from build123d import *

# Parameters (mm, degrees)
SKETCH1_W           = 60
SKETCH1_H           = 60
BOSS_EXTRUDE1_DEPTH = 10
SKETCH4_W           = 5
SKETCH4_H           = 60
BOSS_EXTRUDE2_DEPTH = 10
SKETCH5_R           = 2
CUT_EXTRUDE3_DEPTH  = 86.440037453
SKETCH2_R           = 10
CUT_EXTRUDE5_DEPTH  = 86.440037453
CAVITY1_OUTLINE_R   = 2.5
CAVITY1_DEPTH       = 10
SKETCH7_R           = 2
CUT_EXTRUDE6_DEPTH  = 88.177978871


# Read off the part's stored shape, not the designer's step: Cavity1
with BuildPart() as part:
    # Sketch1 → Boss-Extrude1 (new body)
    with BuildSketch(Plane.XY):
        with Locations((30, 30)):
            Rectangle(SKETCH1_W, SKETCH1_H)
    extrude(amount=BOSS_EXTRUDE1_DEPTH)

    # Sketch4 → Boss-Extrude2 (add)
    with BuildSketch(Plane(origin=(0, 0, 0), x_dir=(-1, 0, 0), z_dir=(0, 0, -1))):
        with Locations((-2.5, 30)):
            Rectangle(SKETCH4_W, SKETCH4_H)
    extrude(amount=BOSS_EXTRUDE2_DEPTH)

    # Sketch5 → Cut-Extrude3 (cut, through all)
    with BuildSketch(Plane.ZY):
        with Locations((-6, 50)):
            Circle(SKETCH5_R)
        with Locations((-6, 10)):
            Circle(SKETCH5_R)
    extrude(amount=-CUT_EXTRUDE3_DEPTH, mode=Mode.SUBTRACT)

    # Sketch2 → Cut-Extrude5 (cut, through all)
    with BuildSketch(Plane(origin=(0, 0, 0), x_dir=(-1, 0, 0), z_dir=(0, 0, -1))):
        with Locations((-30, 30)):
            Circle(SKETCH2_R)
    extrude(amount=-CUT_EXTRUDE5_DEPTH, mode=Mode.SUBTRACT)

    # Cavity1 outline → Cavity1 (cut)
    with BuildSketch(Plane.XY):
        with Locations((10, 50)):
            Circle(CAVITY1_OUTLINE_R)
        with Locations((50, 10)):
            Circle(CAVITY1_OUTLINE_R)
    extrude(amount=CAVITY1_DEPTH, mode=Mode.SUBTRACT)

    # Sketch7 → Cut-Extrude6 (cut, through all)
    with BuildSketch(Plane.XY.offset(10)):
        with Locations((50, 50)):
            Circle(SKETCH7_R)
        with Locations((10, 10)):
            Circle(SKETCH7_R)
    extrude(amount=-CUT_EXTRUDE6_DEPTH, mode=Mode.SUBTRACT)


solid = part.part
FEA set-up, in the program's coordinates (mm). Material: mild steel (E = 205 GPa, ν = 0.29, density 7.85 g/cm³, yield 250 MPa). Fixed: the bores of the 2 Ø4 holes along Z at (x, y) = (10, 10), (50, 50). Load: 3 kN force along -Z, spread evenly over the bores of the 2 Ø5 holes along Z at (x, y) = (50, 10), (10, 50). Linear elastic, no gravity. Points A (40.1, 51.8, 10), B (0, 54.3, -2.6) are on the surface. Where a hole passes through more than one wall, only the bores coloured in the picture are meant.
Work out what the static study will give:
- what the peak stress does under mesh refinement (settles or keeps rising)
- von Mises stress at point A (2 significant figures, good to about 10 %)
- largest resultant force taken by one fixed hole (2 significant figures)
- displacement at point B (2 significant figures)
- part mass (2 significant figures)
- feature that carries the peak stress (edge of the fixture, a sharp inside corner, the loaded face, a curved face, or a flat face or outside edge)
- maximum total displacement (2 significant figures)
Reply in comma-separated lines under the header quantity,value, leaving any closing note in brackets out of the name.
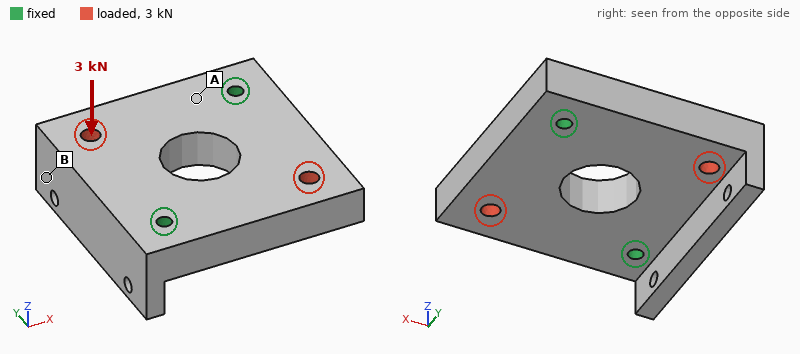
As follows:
quantity,value
what the peak stress does under mesh refinement,keeps rising
von Mises stress at point A,31 MPa
largest resultant force taken by one fixed hole,1.6 kN
displacement at point B,27 µm
part mass,280 g
feature that carries the peak stress,edge of the fixture
maximum total displacement,39 µm
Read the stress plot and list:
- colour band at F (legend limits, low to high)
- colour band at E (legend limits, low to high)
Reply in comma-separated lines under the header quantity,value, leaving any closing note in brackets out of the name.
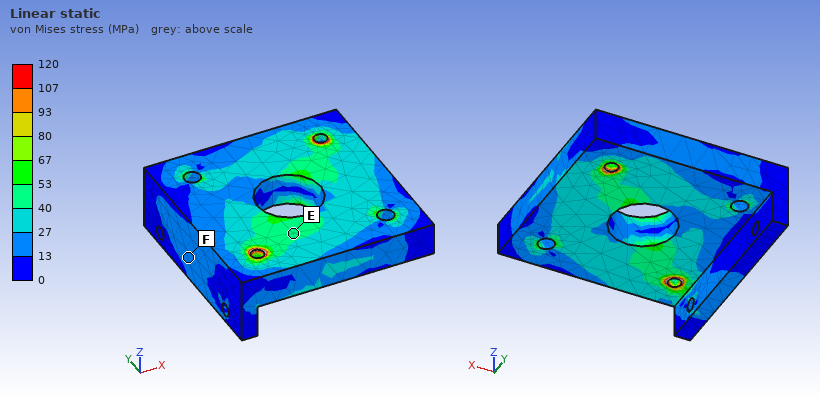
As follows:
quantity,value
colour band at F,13 to 27 MPa
colour band at E,40 to 53 MPa
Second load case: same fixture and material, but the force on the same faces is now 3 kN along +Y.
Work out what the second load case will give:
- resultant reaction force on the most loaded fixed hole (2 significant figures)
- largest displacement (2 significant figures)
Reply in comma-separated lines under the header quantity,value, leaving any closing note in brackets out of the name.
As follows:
quantity,value
resultant reaction force on the most loaded fixed hole,1.5 kN
largest displacement,2.1 µm
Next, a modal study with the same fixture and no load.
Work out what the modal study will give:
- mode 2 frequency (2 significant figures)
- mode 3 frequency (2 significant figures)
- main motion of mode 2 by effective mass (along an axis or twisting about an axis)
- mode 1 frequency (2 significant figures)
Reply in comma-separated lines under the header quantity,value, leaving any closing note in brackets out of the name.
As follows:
quantity,value
mode 2 frequency,5800 Hz
mode 3 frequency,13 kHz
main motion of mode 2 by effective mass,along Z
mode 1 frequency,4500 Hz
